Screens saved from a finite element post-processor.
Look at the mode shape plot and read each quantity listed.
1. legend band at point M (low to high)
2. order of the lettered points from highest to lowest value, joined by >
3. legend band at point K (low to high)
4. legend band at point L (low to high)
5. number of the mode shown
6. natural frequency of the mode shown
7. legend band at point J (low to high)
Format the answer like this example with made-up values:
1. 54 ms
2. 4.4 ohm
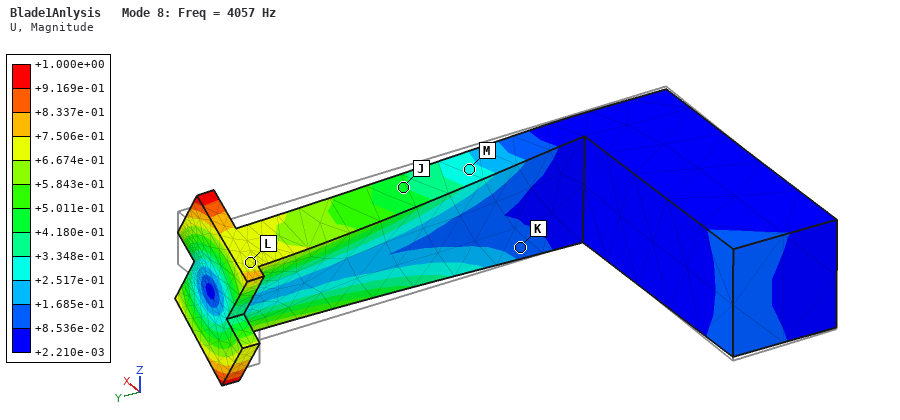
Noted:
1. +2.517e-01 to +3.348e-01
2. L > J > M > K
3. +8.536e-02 to +1.685e-01
4. +6.674e-01 to +7.506e-01
5. 8
6. 4057 Hz
7. +4.180e-01 to +5.011e-01
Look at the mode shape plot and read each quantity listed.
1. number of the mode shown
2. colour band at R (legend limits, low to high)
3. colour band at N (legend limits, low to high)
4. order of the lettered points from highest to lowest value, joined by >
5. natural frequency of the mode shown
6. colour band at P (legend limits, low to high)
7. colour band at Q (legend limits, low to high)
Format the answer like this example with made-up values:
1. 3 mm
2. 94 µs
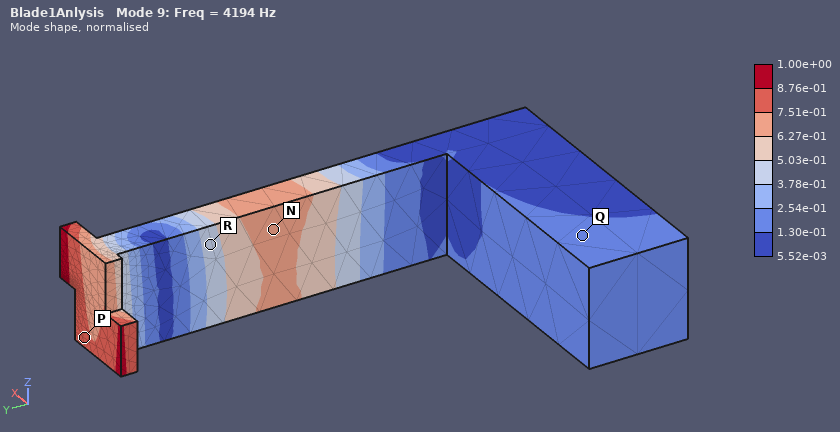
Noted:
1. 9
2. 3.78e-01 to 5.03e-01
3. 6.27e-01 to 7.51e-01
4. P > N > R > Q
5. 4194 Hz
6. 7.51e-01 to 8.76e-01
7. 1.30e-01 to 2.54e-01
